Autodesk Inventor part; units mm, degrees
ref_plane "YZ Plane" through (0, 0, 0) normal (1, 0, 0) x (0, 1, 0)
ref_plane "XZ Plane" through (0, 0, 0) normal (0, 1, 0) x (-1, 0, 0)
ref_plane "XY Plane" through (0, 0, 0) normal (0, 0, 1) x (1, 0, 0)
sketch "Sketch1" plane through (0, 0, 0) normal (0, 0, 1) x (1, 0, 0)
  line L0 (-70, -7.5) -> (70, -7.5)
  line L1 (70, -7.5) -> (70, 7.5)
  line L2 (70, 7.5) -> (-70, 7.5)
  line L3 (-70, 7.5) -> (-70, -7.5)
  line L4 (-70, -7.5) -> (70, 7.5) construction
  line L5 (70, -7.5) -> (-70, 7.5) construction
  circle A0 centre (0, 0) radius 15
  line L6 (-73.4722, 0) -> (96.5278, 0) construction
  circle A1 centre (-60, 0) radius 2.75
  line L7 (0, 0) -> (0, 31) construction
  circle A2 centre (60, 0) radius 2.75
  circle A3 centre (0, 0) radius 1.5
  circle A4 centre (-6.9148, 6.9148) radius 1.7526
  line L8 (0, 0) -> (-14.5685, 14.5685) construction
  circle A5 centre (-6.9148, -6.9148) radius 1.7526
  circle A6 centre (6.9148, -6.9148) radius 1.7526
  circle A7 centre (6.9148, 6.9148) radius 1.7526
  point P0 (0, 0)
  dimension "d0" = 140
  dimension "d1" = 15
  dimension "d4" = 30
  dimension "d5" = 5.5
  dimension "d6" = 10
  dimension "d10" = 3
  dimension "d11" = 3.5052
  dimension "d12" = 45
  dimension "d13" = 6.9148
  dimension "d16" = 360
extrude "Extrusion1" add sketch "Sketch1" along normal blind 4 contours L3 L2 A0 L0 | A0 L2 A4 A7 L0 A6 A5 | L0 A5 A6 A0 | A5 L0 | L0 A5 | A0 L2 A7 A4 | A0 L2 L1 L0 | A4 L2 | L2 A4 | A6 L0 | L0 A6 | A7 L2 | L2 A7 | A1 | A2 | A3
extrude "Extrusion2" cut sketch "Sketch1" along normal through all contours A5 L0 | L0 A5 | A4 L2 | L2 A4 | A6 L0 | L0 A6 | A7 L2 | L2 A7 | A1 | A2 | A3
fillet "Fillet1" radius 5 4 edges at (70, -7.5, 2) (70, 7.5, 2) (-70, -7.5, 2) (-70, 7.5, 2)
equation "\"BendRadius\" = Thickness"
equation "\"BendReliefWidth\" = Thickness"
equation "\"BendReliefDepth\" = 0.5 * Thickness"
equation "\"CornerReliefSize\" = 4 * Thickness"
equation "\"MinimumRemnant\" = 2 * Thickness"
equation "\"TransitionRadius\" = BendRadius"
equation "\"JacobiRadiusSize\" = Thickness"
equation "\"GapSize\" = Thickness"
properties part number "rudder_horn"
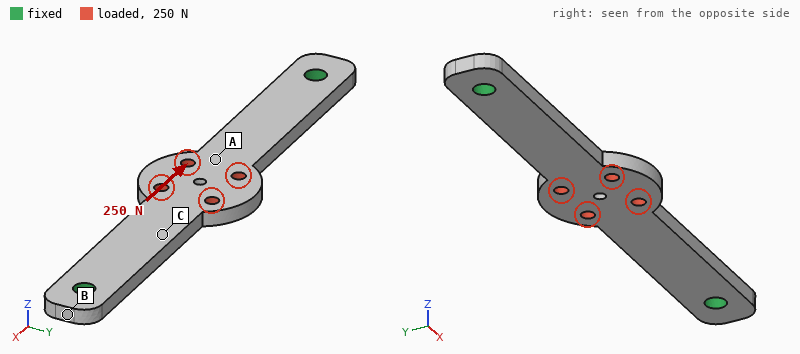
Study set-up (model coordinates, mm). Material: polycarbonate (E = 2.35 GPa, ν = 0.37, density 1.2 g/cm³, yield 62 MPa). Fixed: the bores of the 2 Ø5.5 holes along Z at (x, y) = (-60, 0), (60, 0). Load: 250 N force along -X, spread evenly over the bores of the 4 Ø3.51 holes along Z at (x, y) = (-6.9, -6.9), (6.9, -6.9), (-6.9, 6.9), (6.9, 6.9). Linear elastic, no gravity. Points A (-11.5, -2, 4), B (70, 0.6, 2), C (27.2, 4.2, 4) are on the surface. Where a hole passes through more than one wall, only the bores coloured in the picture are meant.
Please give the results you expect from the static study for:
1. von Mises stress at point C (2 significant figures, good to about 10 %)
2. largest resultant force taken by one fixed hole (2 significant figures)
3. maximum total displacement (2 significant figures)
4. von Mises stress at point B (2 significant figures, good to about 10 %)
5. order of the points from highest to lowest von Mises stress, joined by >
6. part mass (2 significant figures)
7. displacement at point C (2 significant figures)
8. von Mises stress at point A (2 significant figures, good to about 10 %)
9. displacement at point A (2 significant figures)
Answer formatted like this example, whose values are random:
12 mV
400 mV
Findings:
2.1 MPa
130 N
51 µm
0.45 MPa
C > A > B
11 g
29 µm
1.6 MPa
42 µm
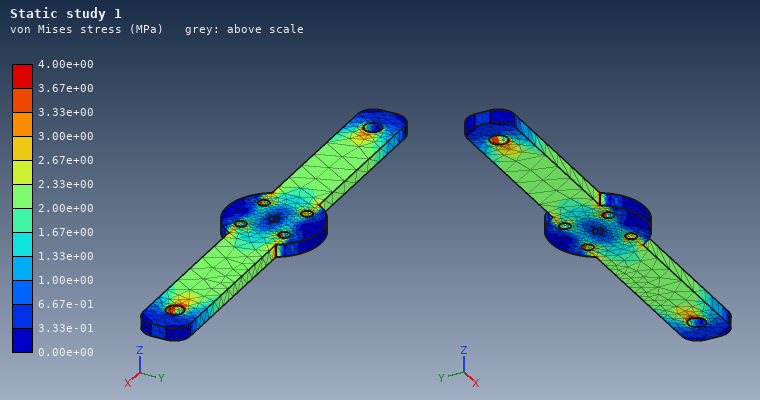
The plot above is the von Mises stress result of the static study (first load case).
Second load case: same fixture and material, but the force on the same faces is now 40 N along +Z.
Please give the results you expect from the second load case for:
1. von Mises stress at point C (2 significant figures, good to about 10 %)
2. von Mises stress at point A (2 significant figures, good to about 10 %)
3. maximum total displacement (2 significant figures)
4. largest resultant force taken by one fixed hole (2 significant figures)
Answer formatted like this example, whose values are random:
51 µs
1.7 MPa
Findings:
1.9 MPa
9.0 MPa
1.6 mm
20 N
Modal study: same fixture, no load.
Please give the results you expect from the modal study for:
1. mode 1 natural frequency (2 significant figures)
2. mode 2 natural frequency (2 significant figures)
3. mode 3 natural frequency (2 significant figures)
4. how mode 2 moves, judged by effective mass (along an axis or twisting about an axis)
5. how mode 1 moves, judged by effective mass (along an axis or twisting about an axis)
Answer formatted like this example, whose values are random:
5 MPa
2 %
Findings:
380 Hz
1000 Hz
1100 Hz
twisting about X
along Z
